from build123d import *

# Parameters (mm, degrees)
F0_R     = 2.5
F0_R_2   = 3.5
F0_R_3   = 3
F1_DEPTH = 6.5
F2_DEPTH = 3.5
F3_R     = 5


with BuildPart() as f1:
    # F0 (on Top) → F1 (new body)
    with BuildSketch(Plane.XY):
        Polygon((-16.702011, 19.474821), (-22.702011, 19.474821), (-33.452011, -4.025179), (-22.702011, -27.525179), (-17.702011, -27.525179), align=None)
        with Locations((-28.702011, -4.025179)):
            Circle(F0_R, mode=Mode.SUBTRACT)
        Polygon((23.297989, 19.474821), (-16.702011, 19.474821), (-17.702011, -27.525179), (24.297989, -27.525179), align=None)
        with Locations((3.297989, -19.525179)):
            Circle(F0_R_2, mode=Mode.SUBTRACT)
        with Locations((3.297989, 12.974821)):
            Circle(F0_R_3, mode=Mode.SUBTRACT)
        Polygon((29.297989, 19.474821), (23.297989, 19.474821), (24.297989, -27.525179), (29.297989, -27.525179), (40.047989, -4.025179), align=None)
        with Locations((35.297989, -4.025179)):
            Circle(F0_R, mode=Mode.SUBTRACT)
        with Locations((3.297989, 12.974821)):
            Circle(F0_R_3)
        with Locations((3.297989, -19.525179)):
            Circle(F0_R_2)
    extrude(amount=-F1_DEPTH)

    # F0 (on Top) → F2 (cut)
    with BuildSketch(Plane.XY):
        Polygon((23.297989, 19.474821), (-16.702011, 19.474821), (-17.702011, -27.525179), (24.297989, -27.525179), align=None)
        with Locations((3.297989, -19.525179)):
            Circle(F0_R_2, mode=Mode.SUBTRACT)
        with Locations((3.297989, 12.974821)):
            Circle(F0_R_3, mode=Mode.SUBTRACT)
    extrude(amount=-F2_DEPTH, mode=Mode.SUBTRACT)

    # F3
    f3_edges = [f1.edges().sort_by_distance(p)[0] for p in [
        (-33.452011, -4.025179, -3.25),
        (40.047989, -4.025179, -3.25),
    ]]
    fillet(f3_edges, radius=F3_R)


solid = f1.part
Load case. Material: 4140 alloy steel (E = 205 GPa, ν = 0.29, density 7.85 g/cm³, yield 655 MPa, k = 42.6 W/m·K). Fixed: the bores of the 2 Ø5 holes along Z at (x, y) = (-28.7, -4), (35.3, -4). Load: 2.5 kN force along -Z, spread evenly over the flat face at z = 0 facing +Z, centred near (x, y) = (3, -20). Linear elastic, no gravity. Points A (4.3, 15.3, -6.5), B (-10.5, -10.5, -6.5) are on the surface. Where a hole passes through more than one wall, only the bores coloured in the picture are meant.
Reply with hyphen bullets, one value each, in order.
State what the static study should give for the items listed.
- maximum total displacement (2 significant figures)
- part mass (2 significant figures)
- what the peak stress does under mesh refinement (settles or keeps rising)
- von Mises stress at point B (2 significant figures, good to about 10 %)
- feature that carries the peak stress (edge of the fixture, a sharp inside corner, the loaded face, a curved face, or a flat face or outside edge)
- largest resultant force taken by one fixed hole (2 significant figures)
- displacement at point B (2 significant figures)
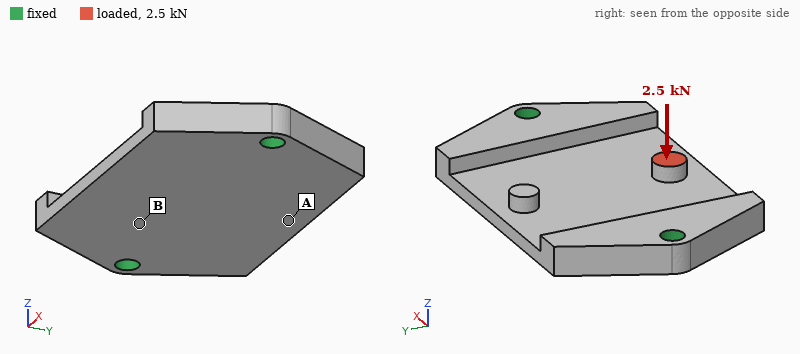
- 0.23 mm
- 97 g
- keeps rising
- 130 MPa
- edge of the fixture
- 2.1 kN
- 0.059 mm
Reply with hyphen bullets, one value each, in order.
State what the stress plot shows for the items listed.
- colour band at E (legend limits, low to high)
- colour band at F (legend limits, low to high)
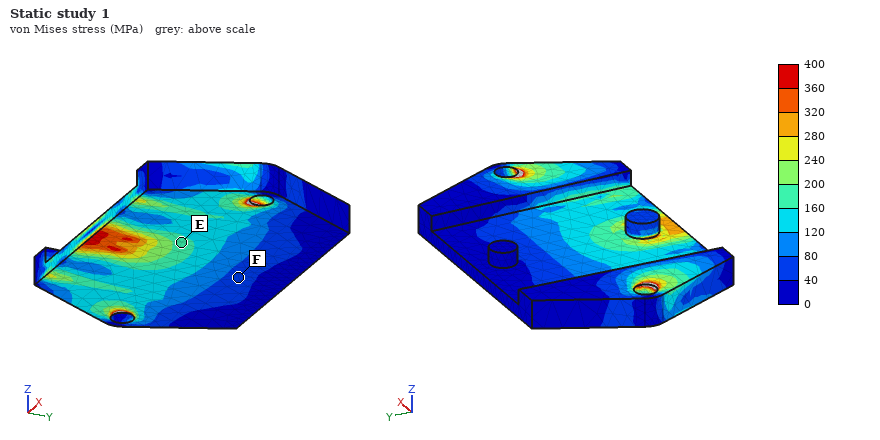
- 160 to 200 MPa
- 40 to 80 MPa
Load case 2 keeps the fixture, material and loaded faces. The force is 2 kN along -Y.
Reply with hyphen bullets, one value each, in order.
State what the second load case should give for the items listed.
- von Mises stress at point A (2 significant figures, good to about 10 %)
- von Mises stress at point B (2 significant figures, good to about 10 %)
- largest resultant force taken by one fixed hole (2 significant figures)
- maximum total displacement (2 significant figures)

- 26 MPa
- 43 MPa
- 1.0 kN
- 66 µm
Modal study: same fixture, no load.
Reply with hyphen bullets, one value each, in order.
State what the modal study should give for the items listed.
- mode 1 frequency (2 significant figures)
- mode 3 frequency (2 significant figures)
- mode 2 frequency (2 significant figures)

- 5200 Hz
- 9100 Hz
- 5400 Hz
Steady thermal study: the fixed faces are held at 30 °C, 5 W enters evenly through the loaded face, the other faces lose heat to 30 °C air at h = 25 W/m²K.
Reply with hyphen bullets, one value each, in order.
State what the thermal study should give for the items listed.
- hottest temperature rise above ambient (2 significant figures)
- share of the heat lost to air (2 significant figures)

- 34 K
- 22 %
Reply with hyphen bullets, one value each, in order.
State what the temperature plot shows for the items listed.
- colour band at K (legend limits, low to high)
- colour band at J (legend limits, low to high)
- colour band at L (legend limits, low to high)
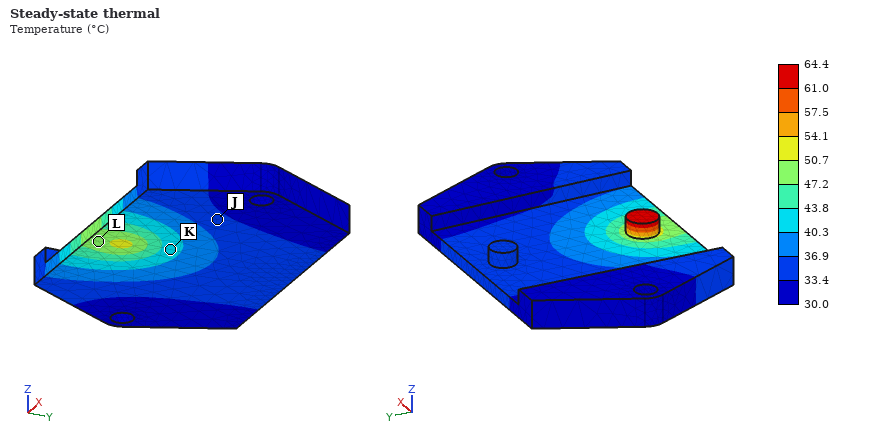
- 40.3 to 43.8 °C
- 33.4 to 36.9 °C
- 47.2 to 50.7 °C
